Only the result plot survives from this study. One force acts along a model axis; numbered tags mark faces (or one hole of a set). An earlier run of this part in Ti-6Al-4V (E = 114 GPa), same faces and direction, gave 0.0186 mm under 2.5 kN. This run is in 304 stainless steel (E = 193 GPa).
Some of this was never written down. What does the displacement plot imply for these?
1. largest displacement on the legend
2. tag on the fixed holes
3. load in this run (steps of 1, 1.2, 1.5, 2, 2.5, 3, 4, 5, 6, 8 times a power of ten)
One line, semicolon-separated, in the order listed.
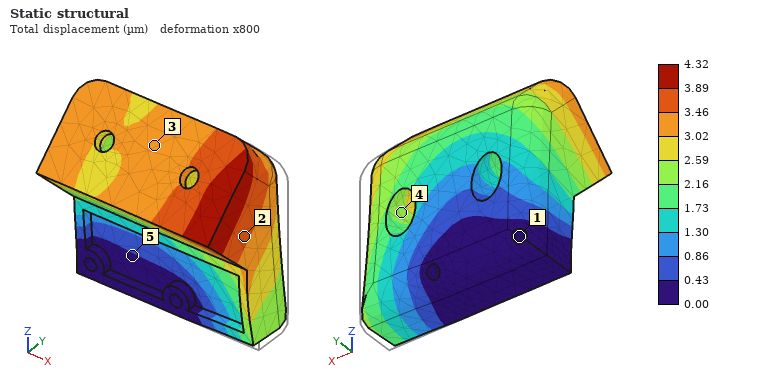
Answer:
4.32 µm; 1; 1 kN
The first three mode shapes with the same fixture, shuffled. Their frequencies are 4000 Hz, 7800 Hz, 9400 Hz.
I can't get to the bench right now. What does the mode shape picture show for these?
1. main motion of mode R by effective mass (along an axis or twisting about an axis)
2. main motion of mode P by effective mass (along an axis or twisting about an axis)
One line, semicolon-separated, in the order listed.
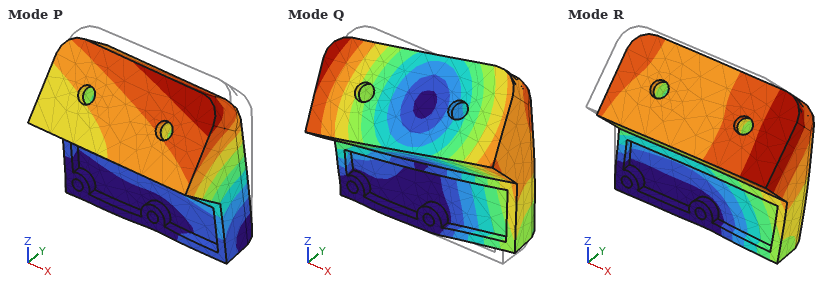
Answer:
along X; along Y
